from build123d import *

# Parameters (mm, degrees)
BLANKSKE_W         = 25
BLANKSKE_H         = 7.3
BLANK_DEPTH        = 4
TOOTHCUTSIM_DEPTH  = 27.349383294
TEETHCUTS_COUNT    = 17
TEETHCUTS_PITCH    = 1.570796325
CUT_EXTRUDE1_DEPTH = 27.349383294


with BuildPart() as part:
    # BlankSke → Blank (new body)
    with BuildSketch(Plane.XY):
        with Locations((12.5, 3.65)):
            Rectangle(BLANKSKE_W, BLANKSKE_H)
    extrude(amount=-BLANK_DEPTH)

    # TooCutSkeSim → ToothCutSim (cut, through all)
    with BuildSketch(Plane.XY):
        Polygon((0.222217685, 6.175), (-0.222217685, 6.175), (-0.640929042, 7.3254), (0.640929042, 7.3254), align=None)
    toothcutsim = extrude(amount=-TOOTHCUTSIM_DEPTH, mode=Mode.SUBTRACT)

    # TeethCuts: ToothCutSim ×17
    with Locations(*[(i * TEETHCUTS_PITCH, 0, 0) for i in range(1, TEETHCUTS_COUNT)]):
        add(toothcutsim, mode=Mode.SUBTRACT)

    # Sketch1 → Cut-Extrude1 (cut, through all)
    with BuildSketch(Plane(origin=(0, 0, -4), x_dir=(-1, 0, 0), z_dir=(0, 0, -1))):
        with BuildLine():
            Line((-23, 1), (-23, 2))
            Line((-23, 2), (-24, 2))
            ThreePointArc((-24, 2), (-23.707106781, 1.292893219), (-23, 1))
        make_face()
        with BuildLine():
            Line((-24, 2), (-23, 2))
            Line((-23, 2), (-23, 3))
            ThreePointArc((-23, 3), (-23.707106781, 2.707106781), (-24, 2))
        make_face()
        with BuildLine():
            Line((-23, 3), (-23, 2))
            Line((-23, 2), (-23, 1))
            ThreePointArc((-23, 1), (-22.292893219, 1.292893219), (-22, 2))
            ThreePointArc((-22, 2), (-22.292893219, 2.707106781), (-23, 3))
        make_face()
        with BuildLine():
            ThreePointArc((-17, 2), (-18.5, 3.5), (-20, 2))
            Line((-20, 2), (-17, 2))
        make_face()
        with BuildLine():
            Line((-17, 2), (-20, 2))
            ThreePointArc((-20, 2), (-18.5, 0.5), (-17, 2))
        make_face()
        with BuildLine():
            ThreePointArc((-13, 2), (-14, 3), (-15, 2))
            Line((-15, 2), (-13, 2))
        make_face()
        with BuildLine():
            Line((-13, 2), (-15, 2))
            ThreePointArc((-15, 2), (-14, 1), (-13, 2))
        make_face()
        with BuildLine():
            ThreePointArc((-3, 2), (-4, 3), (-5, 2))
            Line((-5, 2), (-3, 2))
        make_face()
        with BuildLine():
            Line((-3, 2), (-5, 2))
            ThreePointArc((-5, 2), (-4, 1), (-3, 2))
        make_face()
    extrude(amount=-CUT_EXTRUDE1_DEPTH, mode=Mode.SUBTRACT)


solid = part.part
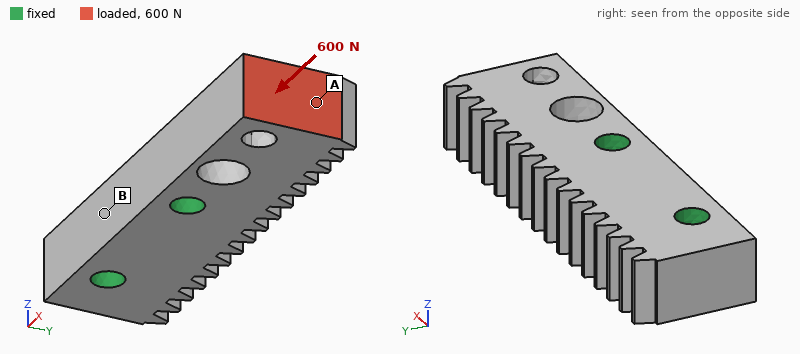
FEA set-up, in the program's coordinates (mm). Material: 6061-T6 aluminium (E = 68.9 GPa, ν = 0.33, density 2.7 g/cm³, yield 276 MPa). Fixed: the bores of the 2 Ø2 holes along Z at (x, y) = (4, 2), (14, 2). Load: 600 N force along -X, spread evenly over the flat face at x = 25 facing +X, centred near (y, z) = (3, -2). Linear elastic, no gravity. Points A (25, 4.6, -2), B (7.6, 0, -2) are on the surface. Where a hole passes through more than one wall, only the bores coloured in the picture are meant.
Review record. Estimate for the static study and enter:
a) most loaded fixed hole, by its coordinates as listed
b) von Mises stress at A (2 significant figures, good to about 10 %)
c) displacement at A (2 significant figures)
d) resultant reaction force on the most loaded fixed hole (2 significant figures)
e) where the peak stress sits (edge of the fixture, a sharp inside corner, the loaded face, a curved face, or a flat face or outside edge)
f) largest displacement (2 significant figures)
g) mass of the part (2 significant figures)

(14, 2)
29 MPa
6.2 µm
520 N
a curved face
8.9 µm
1.6 g
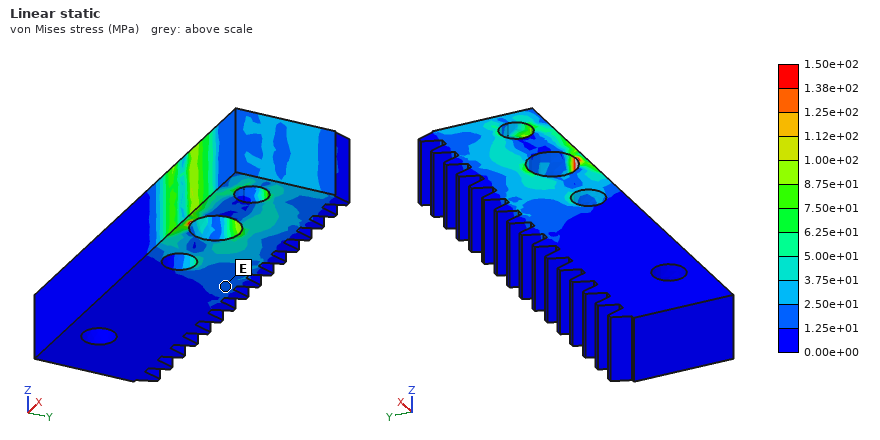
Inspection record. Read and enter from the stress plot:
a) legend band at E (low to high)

1.25e+01 to 2.50e+01 MPa
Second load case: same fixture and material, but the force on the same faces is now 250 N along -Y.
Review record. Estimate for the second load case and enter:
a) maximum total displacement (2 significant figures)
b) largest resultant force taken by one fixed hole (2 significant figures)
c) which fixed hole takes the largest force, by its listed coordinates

48 µm
440 N
(14, 2)
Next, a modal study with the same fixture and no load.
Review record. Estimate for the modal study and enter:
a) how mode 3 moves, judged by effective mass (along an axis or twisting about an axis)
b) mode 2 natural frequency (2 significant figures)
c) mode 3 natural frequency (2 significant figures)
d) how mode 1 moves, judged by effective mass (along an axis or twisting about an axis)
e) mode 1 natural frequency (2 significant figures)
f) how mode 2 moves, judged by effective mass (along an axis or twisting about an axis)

twisting about X
26 kHz
48 kHz
along Z
22 kHz
along Y
